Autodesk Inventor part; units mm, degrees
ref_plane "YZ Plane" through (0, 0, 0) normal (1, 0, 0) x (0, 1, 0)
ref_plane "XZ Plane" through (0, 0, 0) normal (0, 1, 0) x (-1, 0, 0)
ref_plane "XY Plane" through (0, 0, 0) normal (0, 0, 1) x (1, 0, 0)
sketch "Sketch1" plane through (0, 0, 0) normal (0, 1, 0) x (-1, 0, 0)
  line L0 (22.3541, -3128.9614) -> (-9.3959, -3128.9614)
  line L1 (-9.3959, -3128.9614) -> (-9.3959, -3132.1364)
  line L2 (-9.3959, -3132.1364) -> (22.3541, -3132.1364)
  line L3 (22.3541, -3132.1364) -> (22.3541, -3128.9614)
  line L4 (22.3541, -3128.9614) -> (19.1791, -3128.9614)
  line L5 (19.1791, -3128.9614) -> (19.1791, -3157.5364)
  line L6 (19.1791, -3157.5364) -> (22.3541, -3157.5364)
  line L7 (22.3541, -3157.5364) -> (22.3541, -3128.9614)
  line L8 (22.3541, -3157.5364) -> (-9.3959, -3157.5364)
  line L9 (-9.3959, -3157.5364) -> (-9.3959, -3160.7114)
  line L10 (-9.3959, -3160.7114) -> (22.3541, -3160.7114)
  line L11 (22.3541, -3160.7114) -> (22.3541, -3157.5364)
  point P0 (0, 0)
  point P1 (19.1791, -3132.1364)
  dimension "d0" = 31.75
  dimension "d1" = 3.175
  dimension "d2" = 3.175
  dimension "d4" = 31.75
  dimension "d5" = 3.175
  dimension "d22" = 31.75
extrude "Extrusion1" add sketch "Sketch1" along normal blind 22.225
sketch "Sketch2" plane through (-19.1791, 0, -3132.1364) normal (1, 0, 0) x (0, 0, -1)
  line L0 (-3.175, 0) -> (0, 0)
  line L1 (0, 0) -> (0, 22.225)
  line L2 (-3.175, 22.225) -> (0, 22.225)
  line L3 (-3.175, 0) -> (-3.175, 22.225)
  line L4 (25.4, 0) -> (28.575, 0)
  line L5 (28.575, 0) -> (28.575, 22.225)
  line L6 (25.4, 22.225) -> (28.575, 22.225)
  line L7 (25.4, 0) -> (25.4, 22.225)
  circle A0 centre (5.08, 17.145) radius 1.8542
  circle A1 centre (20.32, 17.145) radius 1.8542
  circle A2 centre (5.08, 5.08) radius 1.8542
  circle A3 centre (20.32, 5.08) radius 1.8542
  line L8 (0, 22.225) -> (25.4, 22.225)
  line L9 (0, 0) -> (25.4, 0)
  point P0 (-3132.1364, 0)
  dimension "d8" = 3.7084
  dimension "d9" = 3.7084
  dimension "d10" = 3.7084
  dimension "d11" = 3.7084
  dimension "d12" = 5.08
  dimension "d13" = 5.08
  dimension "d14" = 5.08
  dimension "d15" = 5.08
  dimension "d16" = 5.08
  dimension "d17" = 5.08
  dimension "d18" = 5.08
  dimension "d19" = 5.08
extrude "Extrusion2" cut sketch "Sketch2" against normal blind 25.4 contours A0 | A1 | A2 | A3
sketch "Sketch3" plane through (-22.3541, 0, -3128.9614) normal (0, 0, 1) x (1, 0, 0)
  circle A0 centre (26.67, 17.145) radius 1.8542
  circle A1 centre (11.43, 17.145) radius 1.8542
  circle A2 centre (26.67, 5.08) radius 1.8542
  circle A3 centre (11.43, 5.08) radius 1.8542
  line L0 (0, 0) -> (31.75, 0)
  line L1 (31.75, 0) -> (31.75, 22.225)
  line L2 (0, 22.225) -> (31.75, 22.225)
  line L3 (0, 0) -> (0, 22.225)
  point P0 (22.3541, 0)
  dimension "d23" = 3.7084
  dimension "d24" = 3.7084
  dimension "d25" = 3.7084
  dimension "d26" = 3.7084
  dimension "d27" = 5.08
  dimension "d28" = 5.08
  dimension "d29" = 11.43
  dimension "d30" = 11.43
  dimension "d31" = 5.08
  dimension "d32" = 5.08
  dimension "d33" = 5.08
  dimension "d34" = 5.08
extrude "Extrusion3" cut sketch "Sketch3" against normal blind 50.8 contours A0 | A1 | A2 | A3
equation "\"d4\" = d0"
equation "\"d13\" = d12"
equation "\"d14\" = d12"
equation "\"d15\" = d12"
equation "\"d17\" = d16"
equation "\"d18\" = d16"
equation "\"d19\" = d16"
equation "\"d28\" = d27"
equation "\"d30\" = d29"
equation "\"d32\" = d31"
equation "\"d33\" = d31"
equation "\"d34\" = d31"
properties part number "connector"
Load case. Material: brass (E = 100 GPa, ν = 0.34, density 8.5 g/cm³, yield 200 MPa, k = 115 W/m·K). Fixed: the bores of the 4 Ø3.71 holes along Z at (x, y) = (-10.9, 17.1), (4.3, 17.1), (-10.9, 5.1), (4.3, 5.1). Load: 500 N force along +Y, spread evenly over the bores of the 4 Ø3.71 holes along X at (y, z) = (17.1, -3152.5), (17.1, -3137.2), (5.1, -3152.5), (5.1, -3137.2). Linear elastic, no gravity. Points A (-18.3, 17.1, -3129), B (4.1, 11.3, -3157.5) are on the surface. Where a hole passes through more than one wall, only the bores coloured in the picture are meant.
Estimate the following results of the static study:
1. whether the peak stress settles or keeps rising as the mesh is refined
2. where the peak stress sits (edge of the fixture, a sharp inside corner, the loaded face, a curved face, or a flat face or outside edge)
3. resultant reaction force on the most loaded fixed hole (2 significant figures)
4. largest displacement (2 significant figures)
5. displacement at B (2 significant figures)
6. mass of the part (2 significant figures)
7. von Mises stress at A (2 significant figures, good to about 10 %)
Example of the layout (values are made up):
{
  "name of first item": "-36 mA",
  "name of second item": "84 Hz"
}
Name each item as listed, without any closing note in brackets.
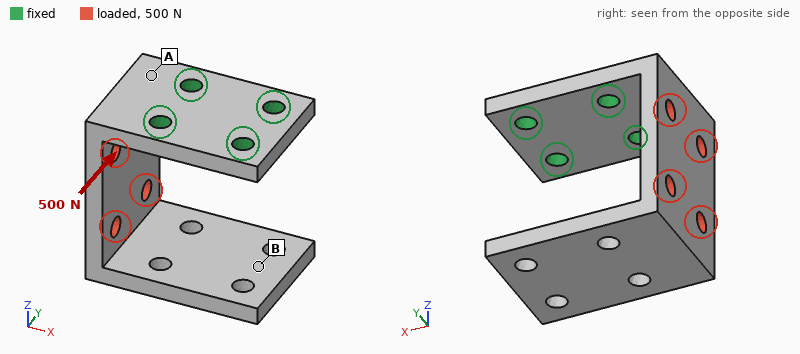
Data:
{
  "whether the peak stress settles or keeps rising as the mesh is refined": "keeps rising",
  "where the peak stress sits": "edge of the fixture",
  "resultant reaction force on the most loaded fixed hole": "610 N",
  "largest displacement": "0.15 mm",
  "displacement at B": "0.12 mm",
  "mass of the part": "50 g",
  "von Mises stress at A": "53 MPa"
}
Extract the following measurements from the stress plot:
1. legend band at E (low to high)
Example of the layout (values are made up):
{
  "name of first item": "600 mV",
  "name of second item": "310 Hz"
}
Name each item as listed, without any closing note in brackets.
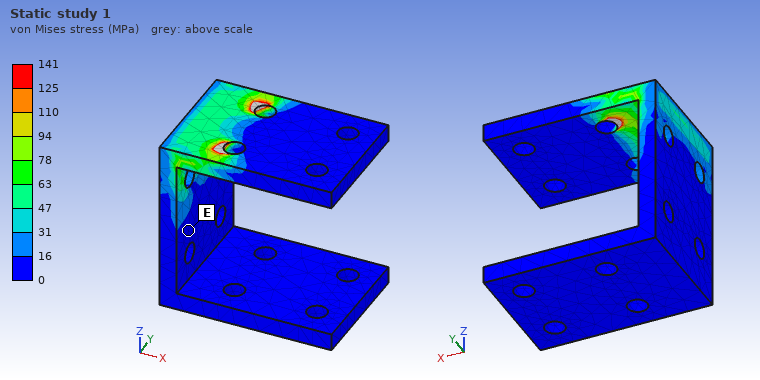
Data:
{
  "legend band at E": "0 to 16 MPa"
}
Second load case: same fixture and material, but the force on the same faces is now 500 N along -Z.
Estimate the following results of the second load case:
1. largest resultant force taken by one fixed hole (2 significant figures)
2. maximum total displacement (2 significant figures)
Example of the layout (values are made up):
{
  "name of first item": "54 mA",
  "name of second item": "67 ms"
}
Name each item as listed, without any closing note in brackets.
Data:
{
  "largest resultant force taken by one fixed hole": "260 N",
  "maximum total displacement": "0.13 mm"
}
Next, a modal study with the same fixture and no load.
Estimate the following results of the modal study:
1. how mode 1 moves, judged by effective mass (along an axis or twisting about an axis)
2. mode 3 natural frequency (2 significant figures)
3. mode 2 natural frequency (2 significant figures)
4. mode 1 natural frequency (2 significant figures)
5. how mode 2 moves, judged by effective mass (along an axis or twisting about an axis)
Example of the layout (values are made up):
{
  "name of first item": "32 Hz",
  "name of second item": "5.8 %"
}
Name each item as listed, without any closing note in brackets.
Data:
{
  "how mode 1 moves, judged by effective mass": "along X",
  "mode 3 natural frequency": "1500 Hz",
  "mode 2 natural frequency": "960 Hz",
  "mode 1 natural frequency": "570 Hz",
  "how mode 2 moves, judged by effective mass": "along Y"
}
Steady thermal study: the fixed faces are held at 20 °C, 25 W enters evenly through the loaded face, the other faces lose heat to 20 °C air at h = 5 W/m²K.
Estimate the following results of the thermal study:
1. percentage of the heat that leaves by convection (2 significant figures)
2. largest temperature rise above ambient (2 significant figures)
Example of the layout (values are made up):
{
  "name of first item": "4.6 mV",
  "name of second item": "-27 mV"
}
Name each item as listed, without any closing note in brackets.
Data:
{
  "percentage of the heat that leaves by convection": "4.0 %",
  "largest temperature rise above ambient": "73 K"
}
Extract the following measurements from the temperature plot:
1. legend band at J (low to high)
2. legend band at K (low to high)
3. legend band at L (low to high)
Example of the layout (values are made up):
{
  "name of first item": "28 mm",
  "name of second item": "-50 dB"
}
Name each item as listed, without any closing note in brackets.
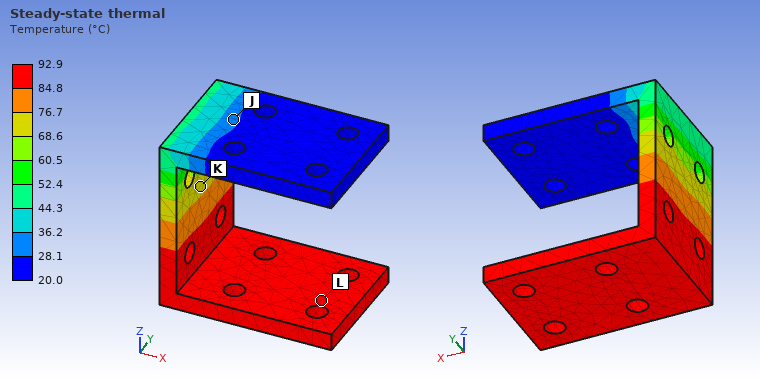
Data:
{
  "legend band at J": "28.1 to 36.2 °C",
  "legend band at K": "68.6 to 76.7 °C",
  "legend band at L": "84.8 to 92.9 °C"
}
